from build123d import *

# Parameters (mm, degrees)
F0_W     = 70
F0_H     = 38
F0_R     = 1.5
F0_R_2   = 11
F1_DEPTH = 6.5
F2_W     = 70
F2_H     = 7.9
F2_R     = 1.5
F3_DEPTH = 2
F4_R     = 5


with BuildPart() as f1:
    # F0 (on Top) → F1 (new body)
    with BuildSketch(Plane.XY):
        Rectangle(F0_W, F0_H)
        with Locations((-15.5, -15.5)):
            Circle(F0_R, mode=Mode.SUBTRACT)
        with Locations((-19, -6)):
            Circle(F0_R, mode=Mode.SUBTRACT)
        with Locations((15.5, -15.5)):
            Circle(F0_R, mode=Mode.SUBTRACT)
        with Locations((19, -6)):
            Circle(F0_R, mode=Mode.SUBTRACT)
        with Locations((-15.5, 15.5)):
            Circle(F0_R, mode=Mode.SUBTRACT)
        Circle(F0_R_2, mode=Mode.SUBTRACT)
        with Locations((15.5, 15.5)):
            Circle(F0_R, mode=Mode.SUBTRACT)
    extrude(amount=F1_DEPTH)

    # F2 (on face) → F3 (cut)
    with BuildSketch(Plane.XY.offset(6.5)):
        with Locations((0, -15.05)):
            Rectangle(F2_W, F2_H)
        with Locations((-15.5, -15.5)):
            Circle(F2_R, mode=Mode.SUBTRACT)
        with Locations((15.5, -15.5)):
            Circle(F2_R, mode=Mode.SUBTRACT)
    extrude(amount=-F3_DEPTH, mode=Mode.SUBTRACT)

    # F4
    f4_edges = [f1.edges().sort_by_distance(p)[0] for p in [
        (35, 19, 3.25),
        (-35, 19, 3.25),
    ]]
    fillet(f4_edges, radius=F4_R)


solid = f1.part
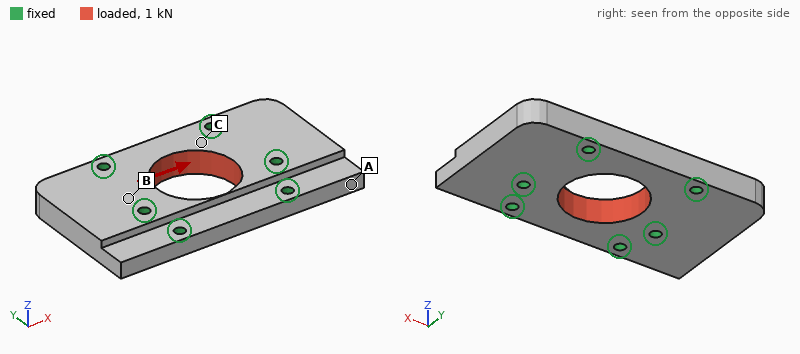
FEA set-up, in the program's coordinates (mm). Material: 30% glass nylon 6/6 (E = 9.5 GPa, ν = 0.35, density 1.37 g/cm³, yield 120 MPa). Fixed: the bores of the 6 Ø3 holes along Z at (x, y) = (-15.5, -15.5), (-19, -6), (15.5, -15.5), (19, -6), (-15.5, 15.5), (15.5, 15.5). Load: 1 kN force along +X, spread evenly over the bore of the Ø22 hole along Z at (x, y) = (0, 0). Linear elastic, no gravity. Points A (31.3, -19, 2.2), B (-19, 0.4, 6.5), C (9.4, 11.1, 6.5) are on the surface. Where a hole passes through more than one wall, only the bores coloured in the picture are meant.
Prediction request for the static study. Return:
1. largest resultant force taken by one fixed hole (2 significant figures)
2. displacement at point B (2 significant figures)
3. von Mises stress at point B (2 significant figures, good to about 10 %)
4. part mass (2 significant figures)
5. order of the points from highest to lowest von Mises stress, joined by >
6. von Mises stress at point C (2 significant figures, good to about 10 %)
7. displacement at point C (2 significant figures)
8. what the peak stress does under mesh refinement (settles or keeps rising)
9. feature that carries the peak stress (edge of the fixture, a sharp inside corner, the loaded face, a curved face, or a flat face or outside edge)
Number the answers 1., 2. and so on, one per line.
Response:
1. 220 N
2. 2.2 µm
3. 1.4 MPa
4. 18 g
5. C > B > A
6. 2.4 MPa
7. 2.4 µm
8. keeps rising
9. a sharp inside corner
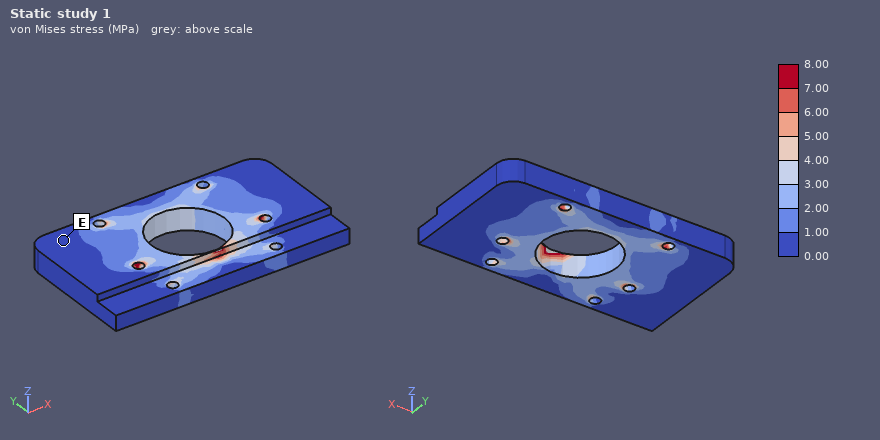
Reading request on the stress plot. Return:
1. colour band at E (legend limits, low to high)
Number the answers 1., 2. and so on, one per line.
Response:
1. 0.00 to 1.00 MPa
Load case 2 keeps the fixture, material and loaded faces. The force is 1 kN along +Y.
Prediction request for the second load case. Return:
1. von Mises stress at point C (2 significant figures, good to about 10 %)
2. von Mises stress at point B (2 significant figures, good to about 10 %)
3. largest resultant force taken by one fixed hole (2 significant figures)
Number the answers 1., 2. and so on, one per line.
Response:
1. 3.5 MPa
2. 1.9 MPa
3. 220 N
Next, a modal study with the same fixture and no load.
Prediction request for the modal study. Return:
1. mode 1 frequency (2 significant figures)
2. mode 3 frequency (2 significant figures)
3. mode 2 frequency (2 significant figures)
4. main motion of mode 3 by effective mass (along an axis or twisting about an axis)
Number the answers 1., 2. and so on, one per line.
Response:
1. 7300 Hz
2. 10 kHz
3. 7400 Hz
4. twisting about X
